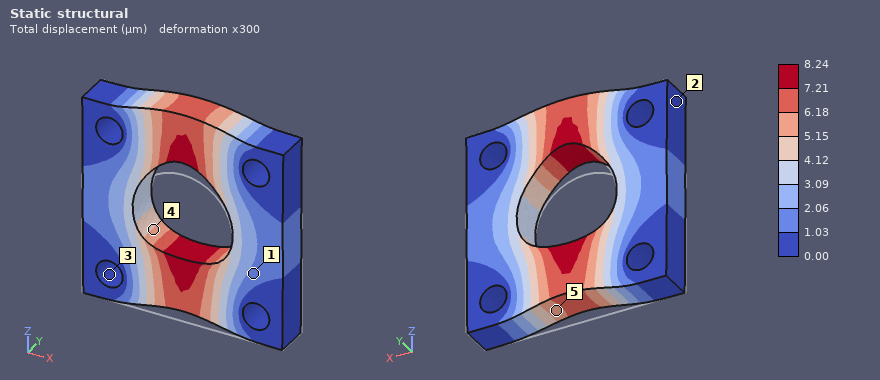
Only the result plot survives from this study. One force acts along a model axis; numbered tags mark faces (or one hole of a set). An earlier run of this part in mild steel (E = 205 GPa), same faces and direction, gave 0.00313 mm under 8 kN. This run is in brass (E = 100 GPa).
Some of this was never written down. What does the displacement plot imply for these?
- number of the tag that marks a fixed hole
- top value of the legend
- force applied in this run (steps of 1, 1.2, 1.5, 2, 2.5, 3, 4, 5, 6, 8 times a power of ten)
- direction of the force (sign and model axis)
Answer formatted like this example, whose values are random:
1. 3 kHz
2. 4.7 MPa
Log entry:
1. 3
2. 8.24 µm
3. 10 kN
4. +Z
